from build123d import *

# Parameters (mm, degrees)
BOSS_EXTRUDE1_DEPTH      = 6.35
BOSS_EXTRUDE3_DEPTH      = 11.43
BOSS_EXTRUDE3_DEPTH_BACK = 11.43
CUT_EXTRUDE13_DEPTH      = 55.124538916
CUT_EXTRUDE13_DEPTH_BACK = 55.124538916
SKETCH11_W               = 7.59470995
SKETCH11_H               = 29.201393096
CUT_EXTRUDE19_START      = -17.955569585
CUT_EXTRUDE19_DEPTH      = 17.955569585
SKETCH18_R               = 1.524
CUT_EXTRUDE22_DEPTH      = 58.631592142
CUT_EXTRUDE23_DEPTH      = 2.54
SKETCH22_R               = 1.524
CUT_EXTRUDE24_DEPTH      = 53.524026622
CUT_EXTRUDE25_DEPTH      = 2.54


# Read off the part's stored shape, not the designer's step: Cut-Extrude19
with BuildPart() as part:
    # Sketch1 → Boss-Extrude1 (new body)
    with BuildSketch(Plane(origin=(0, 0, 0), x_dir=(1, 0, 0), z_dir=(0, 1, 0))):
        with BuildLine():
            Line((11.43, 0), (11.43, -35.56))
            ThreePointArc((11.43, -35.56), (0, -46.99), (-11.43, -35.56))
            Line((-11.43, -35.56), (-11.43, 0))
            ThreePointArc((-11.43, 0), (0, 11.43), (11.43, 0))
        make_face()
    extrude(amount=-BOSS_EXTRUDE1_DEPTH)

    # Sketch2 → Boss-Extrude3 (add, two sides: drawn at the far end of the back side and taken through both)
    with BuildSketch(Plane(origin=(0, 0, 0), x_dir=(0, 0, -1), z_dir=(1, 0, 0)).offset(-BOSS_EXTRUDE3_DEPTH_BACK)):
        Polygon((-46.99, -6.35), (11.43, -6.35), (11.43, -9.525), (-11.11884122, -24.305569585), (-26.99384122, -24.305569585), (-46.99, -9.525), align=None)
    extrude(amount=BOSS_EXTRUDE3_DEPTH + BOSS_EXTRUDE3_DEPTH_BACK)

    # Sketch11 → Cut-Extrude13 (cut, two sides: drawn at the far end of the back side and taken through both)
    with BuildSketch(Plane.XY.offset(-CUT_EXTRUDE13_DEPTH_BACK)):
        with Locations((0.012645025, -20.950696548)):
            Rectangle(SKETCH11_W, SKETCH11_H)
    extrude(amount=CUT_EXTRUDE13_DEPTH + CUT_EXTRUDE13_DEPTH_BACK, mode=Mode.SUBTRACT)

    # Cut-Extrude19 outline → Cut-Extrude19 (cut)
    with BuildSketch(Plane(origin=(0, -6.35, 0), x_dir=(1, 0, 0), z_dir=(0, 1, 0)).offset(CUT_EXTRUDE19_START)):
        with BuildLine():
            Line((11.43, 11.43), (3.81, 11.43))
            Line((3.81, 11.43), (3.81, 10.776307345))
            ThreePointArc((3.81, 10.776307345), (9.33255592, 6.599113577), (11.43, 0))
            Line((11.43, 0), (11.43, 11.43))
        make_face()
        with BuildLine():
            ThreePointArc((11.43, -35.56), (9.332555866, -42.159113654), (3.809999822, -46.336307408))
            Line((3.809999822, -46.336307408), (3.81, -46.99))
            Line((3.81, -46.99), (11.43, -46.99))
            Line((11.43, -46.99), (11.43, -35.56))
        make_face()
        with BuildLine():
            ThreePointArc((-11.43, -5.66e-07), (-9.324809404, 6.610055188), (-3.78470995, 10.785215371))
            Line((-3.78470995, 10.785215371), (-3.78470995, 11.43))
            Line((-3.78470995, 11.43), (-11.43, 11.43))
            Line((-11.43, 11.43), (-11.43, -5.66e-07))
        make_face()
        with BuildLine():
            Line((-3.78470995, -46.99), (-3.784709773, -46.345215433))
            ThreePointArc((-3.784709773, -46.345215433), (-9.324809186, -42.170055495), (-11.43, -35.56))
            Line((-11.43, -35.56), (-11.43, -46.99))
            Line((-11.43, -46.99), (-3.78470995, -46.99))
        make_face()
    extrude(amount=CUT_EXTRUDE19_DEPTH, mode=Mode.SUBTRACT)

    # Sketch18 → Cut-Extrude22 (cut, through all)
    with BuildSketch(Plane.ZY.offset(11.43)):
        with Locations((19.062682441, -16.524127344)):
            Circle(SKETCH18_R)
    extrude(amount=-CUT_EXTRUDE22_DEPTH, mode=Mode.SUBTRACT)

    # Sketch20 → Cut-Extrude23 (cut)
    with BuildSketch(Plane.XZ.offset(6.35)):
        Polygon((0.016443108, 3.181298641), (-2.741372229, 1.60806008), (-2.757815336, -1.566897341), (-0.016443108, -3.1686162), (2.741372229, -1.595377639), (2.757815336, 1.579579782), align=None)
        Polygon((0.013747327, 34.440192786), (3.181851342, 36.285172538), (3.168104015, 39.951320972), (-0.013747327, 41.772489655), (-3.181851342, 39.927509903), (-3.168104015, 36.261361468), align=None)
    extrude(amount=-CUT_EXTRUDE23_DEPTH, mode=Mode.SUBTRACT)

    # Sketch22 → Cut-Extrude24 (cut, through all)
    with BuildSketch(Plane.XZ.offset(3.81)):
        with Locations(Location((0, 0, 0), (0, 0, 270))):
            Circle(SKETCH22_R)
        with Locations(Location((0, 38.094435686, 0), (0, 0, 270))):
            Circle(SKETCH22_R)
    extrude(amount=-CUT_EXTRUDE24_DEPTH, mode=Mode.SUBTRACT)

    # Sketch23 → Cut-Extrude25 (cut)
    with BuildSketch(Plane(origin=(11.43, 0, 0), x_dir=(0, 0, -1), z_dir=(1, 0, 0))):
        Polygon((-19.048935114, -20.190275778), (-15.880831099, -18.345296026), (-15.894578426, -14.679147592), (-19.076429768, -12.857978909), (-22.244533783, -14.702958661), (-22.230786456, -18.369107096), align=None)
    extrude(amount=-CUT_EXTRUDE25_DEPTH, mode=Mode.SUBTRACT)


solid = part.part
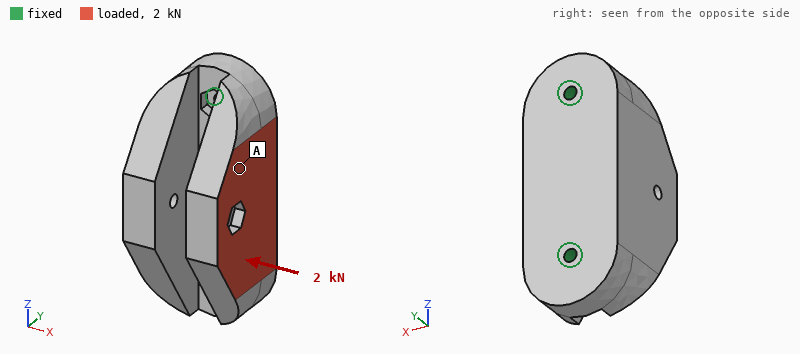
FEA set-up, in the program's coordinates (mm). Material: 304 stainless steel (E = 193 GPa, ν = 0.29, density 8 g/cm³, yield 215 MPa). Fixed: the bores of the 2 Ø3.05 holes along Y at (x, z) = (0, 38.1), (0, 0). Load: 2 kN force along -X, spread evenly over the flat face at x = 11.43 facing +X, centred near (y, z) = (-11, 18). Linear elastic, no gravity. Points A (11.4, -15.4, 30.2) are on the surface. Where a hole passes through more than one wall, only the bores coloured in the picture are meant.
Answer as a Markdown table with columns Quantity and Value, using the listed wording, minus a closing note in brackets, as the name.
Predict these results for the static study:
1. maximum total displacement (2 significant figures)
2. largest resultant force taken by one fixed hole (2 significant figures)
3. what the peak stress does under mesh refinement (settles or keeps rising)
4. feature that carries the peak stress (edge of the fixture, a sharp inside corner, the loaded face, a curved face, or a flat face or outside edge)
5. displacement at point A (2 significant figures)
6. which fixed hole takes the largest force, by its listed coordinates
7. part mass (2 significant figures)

| Quantity | Value |
|---|---|
| maximum total displacement | 47 µm |
| largest resultant force taken by one fixed hole | 1.1 kN |
| what the peak stress does under mesh refinement | keeps rising |
| feature that carries the peak stress | edge of the fixture |
| displacement at point A | 31 µm |
| which fixed hole takes the largest force, by its listed coordinates | (0, 0) |
| part mass | 140 g |
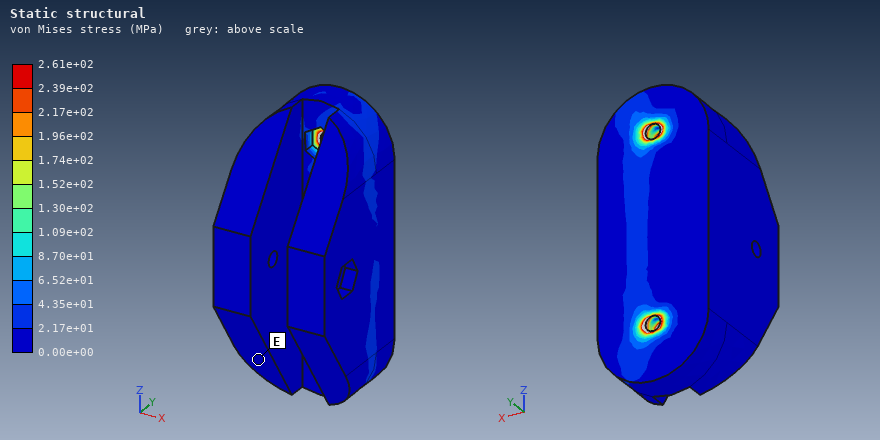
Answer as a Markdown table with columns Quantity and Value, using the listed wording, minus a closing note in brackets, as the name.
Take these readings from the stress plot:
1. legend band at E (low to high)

| Quantity | Value |
|---|---|
| legend band at E | 0.00e+00 to 2.17e+01 MPa |
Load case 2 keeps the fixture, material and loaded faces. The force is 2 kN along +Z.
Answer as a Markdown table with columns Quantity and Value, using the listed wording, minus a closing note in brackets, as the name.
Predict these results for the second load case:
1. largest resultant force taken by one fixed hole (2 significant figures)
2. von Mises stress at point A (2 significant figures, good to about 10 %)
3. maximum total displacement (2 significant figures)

| Quantity | Value |
|---|---|
| largest resultant force taken by one fixed hole | 1.3 kN |
| von Mises stress at point A | 8.0 MPa |
| maximum total displacement | 3.0 µm |
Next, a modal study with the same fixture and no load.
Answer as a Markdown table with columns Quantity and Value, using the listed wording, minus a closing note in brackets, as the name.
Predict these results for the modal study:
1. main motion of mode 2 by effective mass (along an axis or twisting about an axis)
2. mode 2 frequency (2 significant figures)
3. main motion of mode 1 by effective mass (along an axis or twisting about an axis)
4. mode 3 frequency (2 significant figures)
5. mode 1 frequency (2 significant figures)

| Quantity | Value |
|---|---|
| main motion of mode 2 by effective mass | along Y |
| mode 2 frequency | 9400 Hz |
| main motion of mode 1 by effective mass | along X |
| mode 3 frequency | 13 kHz |
| mode 1 frequency | 3900 Hz |
